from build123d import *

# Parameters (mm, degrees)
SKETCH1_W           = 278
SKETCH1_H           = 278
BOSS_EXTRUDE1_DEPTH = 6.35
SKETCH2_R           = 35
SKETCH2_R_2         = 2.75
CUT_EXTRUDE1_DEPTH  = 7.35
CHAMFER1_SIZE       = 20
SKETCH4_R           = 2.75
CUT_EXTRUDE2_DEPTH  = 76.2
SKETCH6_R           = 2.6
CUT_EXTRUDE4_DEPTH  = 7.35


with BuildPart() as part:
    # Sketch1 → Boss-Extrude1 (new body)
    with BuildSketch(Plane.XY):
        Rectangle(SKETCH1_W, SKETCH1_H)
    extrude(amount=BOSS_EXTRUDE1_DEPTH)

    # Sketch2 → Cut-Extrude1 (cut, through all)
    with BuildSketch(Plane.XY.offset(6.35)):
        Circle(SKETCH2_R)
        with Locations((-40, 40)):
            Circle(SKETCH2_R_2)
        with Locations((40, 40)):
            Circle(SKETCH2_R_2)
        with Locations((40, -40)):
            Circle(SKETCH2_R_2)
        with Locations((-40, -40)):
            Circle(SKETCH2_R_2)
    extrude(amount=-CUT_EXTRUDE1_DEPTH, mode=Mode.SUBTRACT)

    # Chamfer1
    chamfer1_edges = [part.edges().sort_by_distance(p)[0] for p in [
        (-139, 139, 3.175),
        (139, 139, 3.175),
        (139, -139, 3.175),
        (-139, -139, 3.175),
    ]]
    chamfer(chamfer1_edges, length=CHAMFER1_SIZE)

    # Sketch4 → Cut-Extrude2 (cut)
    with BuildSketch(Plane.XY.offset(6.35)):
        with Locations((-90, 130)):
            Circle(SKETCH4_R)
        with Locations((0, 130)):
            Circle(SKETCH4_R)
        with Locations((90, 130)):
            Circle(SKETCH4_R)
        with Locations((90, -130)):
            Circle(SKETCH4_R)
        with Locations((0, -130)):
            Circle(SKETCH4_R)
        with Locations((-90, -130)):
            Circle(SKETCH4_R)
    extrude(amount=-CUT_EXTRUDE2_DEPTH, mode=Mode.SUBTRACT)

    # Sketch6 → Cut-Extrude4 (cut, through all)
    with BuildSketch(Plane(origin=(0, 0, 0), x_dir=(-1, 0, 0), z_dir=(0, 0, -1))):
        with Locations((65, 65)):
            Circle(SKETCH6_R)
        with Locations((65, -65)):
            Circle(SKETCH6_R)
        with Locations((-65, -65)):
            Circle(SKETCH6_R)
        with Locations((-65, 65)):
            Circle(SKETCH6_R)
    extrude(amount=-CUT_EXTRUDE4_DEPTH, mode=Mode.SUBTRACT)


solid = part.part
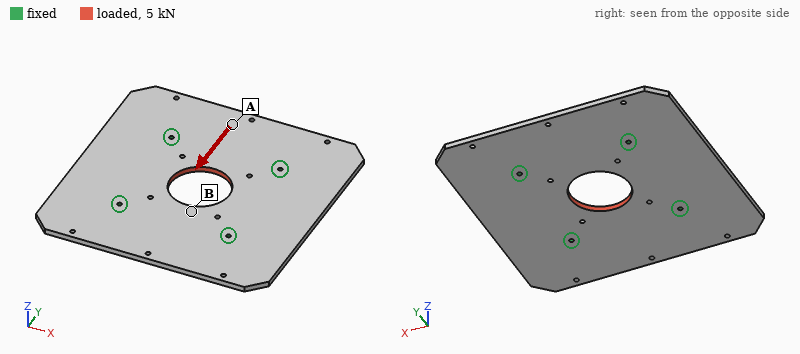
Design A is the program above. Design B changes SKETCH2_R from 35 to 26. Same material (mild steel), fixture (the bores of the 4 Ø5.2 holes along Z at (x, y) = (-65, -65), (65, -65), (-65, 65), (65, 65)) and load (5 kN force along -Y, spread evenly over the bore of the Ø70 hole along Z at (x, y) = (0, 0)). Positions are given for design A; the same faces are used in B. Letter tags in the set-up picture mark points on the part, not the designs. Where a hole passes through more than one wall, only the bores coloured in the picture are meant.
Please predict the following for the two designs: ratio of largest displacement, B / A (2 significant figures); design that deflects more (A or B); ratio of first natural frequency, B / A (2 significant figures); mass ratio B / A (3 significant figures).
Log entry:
1.1
B
1.0
1.02
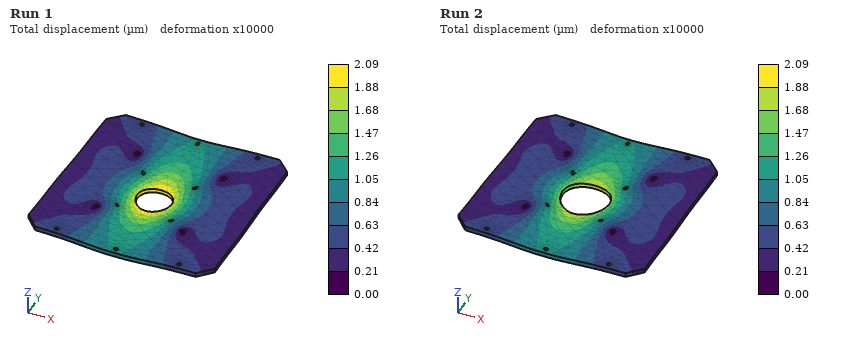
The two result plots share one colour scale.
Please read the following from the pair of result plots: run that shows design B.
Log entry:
Run 1
